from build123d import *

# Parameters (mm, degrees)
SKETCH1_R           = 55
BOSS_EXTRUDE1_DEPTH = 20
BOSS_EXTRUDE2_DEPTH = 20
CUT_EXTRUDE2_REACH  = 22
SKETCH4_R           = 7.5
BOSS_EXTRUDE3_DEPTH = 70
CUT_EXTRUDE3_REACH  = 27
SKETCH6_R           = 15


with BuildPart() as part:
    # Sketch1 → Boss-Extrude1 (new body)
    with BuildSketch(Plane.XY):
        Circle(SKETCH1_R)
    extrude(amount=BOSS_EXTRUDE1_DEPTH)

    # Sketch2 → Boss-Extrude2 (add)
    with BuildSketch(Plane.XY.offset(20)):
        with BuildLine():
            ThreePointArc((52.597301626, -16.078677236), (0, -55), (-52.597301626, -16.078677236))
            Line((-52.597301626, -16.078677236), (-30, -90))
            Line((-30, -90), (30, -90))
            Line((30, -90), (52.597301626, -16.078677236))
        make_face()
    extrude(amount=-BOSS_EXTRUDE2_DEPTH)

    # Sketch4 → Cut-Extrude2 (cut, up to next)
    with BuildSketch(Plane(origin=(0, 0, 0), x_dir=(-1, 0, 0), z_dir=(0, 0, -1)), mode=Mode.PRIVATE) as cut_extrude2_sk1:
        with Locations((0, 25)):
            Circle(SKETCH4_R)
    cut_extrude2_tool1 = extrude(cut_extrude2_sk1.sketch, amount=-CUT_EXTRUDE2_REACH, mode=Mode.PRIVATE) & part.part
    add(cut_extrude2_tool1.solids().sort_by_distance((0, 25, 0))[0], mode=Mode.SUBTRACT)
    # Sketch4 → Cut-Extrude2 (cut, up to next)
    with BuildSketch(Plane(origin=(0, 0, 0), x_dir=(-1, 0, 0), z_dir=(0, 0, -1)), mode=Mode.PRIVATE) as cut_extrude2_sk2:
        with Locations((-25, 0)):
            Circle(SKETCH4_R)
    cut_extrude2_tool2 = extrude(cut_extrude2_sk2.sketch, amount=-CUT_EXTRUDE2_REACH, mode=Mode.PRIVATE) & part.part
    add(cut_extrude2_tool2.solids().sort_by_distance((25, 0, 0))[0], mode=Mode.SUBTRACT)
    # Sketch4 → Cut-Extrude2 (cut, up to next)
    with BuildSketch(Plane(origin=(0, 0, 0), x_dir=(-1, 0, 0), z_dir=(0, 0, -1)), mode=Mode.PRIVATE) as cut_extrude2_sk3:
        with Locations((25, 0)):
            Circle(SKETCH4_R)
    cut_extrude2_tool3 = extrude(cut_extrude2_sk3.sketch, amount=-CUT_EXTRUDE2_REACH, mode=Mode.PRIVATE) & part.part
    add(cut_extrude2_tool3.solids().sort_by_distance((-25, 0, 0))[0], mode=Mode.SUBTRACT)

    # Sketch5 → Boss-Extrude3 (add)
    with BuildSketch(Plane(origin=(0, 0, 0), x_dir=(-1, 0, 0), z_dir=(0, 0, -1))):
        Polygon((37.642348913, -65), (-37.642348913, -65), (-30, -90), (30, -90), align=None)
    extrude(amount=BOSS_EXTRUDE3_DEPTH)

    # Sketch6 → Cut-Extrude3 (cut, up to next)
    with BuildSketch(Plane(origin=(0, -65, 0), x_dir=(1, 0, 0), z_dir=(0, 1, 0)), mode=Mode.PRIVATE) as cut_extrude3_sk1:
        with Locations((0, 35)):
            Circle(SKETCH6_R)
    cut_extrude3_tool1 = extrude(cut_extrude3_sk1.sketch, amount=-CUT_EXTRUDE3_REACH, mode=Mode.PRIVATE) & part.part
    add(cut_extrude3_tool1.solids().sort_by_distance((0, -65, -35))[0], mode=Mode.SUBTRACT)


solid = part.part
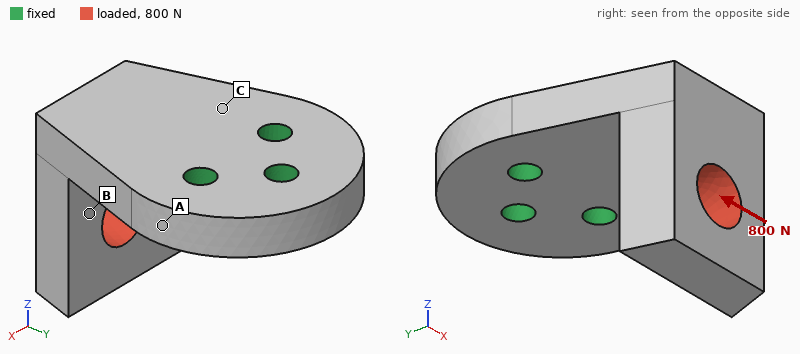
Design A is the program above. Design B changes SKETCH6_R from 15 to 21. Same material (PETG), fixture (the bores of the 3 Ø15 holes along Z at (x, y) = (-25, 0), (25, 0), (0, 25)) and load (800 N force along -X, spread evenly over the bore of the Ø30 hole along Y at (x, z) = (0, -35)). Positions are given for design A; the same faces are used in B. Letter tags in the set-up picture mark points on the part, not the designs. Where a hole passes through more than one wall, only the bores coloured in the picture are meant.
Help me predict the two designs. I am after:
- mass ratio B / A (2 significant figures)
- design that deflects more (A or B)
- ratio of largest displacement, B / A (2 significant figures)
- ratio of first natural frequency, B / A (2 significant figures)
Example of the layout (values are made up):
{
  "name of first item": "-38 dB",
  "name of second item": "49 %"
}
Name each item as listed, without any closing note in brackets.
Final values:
{
  "mass ratio B / A": "0.95",
  "design that deflects more": "B",
  "ratio of largest displacement, B / A": "1.1",
  "ratio of first natural frequency, B / A": "1.1"
}
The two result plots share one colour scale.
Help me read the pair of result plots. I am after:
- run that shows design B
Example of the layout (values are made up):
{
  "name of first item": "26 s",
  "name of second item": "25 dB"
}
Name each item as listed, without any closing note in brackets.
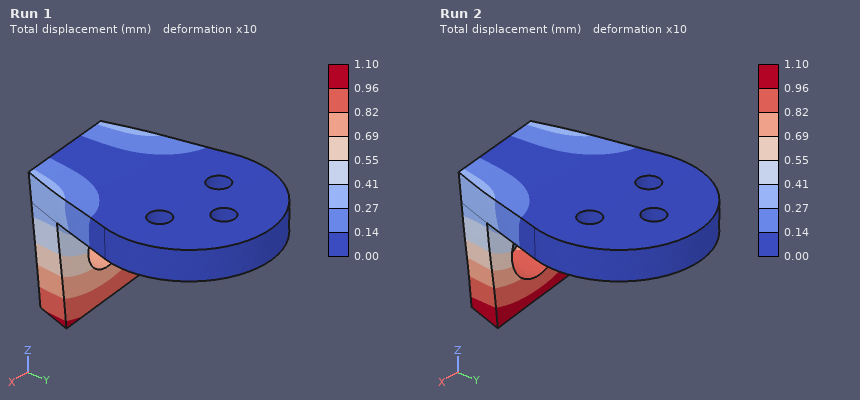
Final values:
{
  "run that shows design B": "Run 2"
}
